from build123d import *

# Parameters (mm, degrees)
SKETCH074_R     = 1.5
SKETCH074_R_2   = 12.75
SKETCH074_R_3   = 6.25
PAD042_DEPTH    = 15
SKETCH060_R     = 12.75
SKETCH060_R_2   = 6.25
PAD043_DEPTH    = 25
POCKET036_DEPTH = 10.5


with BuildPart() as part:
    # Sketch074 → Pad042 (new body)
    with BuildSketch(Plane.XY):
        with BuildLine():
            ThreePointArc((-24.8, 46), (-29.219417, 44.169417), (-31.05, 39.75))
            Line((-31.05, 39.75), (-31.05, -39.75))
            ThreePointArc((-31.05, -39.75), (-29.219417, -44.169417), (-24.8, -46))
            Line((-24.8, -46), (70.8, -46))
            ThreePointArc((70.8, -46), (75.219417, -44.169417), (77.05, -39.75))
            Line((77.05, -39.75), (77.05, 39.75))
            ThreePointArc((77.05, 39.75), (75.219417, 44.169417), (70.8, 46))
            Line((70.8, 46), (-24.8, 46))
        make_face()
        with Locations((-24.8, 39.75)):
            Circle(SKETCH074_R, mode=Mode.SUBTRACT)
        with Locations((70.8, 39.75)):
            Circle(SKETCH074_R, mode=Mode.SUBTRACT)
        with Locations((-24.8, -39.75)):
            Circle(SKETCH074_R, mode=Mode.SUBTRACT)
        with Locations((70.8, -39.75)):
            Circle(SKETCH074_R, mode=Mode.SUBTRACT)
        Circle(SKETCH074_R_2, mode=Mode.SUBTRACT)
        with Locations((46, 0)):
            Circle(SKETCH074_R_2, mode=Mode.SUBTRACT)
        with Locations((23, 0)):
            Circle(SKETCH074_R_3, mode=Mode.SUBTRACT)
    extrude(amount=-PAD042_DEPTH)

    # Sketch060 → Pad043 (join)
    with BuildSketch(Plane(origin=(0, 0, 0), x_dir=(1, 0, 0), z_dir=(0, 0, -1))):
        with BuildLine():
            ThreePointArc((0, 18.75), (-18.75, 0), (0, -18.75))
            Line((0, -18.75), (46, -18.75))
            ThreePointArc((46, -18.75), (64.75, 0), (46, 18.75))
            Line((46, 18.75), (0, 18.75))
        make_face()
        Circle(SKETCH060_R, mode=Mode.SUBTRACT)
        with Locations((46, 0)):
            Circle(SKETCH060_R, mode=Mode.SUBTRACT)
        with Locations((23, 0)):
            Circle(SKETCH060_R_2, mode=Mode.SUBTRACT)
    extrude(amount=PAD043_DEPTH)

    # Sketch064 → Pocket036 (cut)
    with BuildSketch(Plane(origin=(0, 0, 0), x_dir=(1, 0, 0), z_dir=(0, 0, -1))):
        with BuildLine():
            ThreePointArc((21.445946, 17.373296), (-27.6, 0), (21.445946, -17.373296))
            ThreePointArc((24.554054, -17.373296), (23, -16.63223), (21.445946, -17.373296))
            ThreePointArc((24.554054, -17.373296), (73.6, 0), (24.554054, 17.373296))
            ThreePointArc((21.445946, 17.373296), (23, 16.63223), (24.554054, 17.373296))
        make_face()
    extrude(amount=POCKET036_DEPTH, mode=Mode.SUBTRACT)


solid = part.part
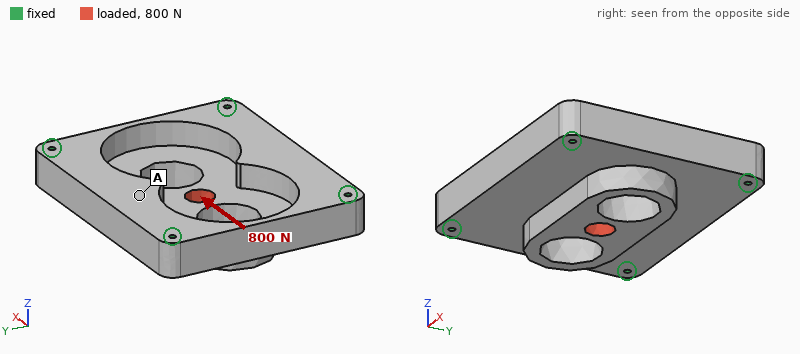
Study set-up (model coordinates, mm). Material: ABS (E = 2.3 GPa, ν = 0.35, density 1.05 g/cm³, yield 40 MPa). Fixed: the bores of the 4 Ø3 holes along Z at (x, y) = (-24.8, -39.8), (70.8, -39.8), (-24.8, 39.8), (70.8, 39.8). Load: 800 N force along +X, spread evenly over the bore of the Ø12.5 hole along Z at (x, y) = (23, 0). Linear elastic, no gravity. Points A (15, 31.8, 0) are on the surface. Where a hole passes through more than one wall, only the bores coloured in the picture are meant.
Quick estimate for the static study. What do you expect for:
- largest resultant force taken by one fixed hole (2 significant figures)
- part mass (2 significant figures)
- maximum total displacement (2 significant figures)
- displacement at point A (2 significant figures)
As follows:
230 N
120 g
60 µm
9.2 µm
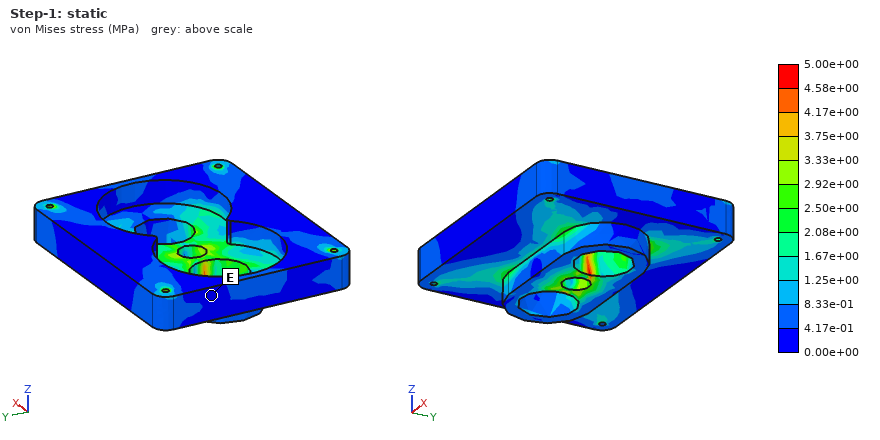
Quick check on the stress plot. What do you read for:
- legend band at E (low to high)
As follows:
0.00e+00 to 4.17e-01 MPa
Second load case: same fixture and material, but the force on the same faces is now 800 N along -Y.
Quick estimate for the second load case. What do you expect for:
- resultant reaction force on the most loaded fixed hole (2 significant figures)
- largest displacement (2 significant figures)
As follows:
260 N
70 µm
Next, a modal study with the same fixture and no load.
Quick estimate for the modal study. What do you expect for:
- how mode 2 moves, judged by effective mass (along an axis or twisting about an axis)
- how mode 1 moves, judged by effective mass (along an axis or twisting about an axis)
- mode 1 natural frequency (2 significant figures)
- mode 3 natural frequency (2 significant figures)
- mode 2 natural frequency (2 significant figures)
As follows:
twisting about X
along Z
1600 Hz
2400 Hz
1900 Hz
